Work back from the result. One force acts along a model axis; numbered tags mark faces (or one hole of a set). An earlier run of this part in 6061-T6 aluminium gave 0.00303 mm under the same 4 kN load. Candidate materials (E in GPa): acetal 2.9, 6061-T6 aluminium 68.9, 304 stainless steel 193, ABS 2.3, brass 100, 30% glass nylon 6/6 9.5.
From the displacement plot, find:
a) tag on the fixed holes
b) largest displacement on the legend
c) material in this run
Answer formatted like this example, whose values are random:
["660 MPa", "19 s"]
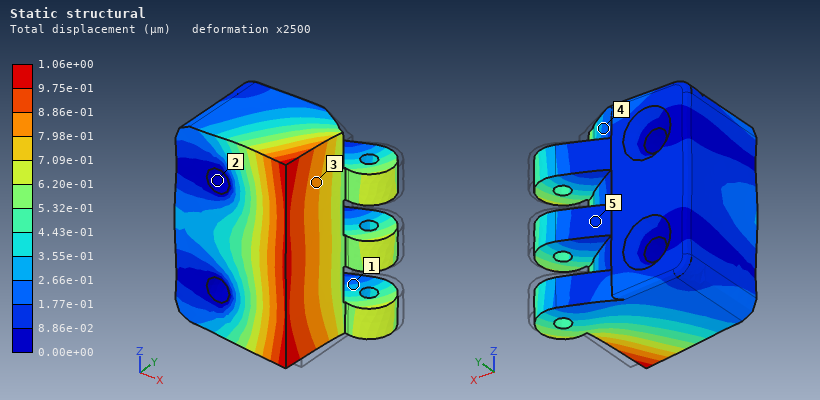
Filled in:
["2", "1.06e+00 µm", "304 stainless steel"]
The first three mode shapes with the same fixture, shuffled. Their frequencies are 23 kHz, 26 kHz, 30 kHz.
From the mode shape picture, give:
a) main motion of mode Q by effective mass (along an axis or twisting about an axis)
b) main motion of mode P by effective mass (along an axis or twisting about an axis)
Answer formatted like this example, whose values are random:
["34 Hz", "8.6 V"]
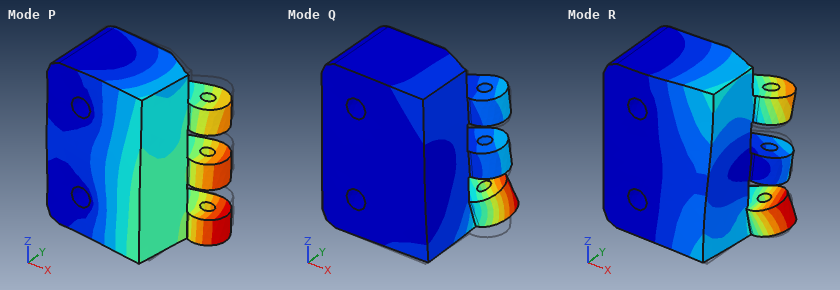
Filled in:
["along Z", "along Y"]
